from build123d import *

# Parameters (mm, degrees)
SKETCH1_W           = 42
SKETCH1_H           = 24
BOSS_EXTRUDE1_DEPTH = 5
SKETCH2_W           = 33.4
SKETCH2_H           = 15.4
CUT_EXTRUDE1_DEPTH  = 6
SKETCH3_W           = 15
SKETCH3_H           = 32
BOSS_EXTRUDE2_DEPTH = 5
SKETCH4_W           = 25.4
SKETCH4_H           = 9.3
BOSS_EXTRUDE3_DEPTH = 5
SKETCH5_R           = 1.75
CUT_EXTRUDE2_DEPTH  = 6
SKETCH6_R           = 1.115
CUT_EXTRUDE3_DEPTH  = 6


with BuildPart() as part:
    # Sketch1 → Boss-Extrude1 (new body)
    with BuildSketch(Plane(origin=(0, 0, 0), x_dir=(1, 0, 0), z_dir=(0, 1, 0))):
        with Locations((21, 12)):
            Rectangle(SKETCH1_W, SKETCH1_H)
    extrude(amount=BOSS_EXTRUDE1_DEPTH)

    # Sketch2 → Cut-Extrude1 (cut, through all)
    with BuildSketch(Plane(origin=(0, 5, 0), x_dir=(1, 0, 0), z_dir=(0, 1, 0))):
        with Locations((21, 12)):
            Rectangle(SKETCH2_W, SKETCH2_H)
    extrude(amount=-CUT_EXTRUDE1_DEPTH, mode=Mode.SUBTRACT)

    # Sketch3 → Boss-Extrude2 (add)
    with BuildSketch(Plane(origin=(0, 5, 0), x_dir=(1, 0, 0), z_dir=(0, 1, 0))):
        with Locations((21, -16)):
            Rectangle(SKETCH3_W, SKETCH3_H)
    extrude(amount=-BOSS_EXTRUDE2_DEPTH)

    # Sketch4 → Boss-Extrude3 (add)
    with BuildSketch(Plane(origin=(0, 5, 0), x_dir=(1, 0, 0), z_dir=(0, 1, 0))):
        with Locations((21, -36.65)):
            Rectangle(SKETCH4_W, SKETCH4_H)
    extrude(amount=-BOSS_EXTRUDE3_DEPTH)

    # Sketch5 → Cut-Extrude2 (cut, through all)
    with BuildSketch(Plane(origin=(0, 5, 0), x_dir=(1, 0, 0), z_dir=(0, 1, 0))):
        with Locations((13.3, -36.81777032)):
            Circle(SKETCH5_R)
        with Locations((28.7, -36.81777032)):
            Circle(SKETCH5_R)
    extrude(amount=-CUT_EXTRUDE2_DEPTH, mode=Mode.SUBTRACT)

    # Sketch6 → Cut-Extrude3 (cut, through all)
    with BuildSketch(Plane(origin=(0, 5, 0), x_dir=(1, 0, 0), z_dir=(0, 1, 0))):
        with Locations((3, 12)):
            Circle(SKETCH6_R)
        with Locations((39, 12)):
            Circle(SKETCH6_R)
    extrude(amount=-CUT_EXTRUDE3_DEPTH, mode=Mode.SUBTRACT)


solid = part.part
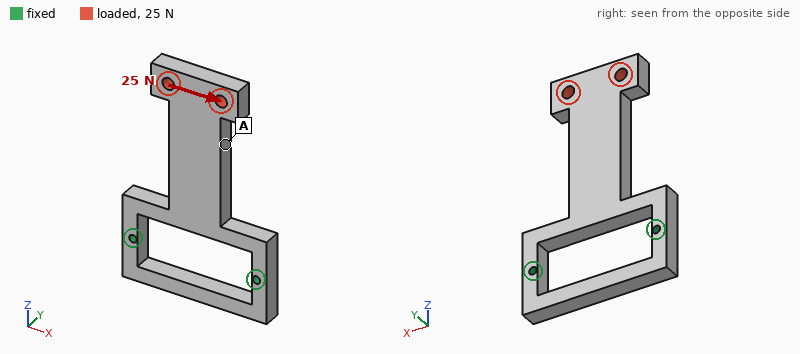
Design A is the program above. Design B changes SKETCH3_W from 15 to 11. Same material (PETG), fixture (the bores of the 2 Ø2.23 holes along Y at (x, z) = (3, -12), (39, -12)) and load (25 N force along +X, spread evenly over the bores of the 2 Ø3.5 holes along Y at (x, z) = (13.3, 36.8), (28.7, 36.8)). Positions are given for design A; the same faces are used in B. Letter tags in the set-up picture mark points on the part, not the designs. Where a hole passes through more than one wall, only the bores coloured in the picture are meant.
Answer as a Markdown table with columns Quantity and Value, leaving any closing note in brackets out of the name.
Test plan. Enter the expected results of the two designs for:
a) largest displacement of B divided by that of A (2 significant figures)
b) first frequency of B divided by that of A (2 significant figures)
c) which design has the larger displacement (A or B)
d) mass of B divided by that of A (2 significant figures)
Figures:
| Quantity | Value |
|---|---|
| largest displacement of B divided by that of A | 1.8 |
| first frequency of B divided by that of A | 0.99 |
| which design has the larger displacement | B |
| mass of B divided by that of A | 0.89 |
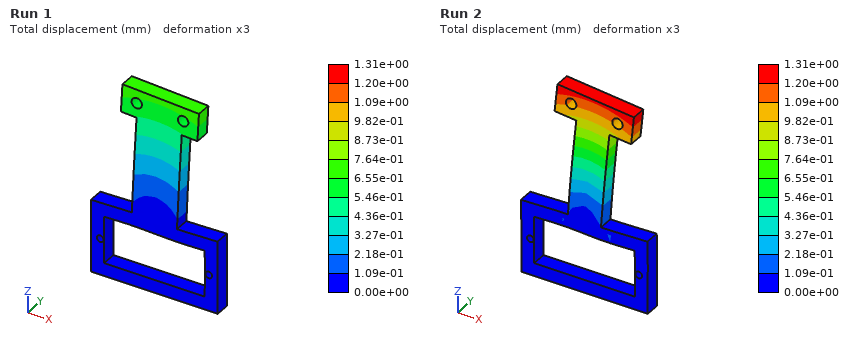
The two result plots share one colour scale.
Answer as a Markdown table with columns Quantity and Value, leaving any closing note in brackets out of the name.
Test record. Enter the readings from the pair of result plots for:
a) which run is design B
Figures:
| Quantity | Value |
|---|---|
| which run is design B | Run 2 |
